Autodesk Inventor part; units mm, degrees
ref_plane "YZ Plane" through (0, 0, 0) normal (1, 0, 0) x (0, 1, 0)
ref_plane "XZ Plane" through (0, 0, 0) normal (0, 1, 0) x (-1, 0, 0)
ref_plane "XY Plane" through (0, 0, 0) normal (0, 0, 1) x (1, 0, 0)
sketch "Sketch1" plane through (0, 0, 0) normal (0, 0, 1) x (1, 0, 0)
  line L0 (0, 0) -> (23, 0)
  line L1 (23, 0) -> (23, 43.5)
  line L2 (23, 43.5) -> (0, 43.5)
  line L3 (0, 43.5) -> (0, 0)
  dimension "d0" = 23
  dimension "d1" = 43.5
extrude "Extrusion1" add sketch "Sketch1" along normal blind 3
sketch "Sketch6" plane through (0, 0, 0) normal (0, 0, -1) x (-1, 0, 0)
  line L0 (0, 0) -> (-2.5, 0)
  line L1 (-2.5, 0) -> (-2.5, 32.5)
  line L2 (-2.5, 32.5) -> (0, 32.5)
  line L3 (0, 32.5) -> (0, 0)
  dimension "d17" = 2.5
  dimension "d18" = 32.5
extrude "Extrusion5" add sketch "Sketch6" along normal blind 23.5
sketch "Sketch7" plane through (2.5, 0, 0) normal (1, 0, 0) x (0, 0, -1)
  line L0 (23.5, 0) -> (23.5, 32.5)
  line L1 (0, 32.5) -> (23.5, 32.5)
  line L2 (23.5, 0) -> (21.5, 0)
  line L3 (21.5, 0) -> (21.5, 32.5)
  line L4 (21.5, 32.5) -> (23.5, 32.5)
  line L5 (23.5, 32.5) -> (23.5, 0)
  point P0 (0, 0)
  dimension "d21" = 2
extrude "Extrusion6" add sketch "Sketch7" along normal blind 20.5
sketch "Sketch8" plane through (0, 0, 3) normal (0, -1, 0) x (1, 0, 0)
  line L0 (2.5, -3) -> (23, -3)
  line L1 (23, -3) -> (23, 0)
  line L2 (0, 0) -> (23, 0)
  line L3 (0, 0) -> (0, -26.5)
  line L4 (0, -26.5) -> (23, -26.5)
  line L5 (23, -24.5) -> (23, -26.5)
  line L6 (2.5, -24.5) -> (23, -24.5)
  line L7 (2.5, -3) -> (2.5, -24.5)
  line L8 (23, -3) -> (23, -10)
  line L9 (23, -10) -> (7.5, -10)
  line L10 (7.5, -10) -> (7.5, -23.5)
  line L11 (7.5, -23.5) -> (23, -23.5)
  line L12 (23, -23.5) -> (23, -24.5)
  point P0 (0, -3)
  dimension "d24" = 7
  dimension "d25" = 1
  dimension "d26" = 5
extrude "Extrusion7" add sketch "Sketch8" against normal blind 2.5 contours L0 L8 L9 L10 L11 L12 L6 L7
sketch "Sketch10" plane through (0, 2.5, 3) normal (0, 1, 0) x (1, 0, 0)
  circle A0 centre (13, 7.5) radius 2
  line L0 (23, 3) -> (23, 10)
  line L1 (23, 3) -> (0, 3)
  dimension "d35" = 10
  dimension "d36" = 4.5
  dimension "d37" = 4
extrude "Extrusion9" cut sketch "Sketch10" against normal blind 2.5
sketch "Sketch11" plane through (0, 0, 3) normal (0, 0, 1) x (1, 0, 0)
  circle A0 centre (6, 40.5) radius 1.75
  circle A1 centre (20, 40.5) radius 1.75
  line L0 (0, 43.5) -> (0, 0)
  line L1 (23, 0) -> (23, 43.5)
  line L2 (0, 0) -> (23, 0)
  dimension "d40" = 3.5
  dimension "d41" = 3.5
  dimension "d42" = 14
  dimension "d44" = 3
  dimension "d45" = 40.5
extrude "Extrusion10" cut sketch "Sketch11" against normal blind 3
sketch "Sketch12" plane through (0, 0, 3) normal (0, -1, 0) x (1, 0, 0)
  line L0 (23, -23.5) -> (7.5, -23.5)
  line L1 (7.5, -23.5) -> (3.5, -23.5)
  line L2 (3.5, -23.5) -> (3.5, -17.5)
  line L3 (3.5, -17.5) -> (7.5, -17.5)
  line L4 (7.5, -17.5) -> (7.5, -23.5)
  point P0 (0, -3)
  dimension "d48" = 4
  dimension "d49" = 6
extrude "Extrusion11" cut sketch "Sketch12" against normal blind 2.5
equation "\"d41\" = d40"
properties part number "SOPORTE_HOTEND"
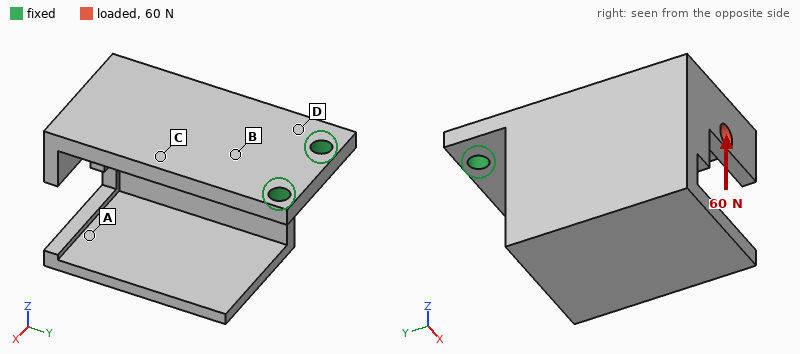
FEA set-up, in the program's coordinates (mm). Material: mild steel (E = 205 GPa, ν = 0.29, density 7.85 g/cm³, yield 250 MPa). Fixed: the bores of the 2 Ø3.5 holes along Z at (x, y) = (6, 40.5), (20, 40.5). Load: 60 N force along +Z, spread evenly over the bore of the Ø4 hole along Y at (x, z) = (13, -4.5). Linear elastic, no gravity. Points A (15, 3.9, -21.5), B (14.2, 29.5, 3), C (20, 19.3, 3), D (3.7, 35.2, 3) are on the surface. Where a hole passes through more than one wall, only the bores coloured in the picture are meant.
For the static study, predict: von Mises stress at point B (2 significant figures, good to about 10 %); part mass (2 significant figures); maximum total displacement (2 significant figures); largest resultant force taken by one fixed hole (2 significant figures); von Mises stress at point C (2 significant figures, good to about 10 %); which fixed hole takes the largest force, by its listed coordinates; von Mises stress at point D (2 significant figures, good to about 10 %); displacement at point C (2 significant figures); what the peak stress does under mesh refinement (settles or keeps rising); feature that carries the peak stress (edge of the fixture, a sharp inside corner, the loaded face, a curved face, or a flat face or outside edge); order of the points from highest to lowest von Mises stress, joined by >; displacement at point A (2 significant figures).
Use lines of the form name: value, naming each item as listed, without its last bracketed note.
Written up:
von Mises stress at point B: 35 MPa
part mass: 52 g
maximum total displacement: 0.10 mm
largest resultant force taken by one fixed hole: 39 N
von Mises stress at point C: 14 MPa
which fixed hole takes the largest force, by its listed coordinates: (6, 40.5)
von Mises stress at point D: 66 MPa
displacement at point C: 0.032 mm
what the peak stress does under mesh refinement: keeps rising
feature that carries the peak stress: edge of the fixture
order of the points from highest to lowest von Mises stress, joined by >: D > B > C > A
displacement at point A: 0.092 mm
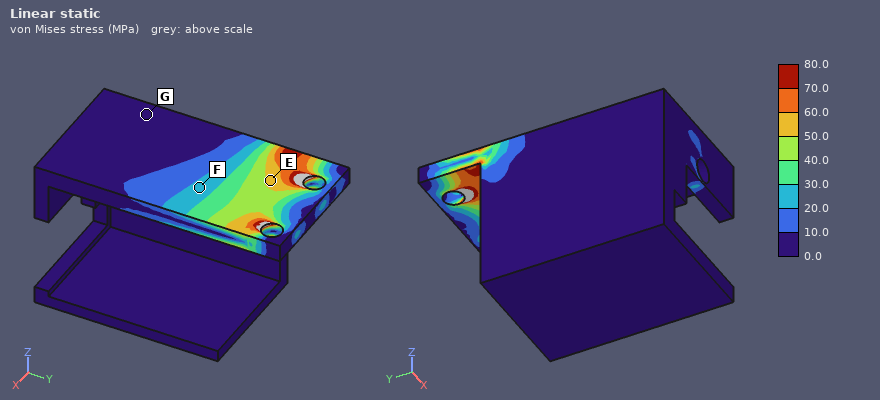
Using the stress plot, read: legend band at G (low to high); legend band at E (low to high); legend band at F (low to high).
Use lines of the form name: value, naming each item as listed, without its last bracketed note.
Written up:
legend band at G: 0.0 to 10.0 MPa
legend band at E: 50.0 to 60.0 MPa
legend band at F: 20.0 to 30.0 MPa
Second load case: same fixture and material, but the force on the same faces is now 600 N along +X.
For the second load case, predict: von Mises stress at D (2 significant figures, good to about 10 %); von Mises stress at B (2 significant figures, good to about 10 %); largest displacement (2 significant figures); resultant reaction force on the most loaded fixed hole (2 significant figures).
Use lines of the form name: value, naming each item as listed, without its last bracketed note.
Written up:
von Mises stress at D: 110 MPa
von Mises stress at B: 42 MPa
largest displacement: 0.18 mm
resultant reaction force on the most loaded fixed hole: 1.5 kN
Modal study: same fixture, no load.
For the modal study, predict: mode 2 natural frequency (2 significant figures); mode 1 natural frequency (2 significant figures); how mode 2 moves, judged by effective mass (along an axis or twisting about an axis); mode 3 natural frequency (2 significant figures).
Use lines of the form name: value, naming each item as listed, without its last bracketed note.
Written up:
mode 2 natural frequency: 1200 Hz
mode 1 natural frequency: 780 Hz
how mode 2 moves, judged by effective mass: along X
mode 3 natural frequency: 2700 Hz
